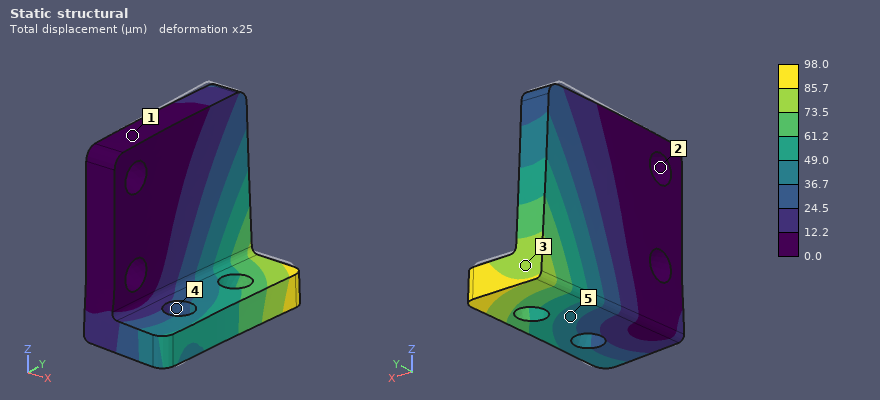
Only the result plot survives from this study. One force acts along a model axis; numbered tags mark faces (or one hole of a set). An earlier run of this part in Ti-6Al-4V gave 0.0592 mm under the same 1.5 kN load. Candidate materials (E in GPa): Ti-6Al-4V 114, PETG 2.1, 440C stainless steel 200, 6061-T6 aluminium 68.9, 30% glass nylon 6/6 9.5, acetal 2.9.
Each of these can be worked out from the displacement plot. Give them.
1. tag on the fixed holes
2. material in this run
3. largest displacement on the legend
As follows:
2
6061-T6 aluminium
98.0 µm
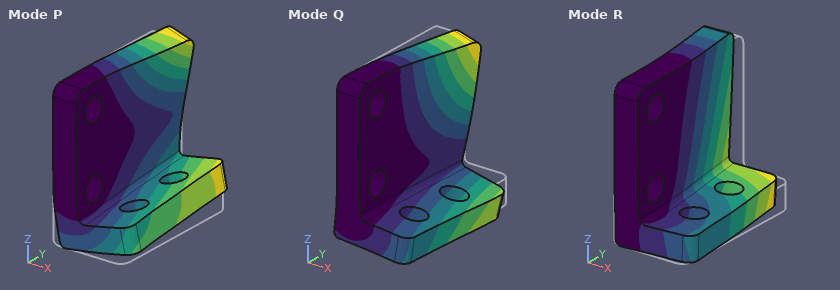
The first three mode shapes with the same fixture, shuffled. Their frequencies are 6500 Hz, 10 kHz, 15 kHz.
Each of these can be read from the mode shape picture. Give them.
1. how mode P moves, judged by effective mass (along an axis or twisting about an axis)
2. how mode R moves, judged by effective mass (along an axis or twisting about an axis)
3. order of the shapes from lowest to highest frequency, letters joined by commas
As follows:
along Z
along X
R, Q, P
